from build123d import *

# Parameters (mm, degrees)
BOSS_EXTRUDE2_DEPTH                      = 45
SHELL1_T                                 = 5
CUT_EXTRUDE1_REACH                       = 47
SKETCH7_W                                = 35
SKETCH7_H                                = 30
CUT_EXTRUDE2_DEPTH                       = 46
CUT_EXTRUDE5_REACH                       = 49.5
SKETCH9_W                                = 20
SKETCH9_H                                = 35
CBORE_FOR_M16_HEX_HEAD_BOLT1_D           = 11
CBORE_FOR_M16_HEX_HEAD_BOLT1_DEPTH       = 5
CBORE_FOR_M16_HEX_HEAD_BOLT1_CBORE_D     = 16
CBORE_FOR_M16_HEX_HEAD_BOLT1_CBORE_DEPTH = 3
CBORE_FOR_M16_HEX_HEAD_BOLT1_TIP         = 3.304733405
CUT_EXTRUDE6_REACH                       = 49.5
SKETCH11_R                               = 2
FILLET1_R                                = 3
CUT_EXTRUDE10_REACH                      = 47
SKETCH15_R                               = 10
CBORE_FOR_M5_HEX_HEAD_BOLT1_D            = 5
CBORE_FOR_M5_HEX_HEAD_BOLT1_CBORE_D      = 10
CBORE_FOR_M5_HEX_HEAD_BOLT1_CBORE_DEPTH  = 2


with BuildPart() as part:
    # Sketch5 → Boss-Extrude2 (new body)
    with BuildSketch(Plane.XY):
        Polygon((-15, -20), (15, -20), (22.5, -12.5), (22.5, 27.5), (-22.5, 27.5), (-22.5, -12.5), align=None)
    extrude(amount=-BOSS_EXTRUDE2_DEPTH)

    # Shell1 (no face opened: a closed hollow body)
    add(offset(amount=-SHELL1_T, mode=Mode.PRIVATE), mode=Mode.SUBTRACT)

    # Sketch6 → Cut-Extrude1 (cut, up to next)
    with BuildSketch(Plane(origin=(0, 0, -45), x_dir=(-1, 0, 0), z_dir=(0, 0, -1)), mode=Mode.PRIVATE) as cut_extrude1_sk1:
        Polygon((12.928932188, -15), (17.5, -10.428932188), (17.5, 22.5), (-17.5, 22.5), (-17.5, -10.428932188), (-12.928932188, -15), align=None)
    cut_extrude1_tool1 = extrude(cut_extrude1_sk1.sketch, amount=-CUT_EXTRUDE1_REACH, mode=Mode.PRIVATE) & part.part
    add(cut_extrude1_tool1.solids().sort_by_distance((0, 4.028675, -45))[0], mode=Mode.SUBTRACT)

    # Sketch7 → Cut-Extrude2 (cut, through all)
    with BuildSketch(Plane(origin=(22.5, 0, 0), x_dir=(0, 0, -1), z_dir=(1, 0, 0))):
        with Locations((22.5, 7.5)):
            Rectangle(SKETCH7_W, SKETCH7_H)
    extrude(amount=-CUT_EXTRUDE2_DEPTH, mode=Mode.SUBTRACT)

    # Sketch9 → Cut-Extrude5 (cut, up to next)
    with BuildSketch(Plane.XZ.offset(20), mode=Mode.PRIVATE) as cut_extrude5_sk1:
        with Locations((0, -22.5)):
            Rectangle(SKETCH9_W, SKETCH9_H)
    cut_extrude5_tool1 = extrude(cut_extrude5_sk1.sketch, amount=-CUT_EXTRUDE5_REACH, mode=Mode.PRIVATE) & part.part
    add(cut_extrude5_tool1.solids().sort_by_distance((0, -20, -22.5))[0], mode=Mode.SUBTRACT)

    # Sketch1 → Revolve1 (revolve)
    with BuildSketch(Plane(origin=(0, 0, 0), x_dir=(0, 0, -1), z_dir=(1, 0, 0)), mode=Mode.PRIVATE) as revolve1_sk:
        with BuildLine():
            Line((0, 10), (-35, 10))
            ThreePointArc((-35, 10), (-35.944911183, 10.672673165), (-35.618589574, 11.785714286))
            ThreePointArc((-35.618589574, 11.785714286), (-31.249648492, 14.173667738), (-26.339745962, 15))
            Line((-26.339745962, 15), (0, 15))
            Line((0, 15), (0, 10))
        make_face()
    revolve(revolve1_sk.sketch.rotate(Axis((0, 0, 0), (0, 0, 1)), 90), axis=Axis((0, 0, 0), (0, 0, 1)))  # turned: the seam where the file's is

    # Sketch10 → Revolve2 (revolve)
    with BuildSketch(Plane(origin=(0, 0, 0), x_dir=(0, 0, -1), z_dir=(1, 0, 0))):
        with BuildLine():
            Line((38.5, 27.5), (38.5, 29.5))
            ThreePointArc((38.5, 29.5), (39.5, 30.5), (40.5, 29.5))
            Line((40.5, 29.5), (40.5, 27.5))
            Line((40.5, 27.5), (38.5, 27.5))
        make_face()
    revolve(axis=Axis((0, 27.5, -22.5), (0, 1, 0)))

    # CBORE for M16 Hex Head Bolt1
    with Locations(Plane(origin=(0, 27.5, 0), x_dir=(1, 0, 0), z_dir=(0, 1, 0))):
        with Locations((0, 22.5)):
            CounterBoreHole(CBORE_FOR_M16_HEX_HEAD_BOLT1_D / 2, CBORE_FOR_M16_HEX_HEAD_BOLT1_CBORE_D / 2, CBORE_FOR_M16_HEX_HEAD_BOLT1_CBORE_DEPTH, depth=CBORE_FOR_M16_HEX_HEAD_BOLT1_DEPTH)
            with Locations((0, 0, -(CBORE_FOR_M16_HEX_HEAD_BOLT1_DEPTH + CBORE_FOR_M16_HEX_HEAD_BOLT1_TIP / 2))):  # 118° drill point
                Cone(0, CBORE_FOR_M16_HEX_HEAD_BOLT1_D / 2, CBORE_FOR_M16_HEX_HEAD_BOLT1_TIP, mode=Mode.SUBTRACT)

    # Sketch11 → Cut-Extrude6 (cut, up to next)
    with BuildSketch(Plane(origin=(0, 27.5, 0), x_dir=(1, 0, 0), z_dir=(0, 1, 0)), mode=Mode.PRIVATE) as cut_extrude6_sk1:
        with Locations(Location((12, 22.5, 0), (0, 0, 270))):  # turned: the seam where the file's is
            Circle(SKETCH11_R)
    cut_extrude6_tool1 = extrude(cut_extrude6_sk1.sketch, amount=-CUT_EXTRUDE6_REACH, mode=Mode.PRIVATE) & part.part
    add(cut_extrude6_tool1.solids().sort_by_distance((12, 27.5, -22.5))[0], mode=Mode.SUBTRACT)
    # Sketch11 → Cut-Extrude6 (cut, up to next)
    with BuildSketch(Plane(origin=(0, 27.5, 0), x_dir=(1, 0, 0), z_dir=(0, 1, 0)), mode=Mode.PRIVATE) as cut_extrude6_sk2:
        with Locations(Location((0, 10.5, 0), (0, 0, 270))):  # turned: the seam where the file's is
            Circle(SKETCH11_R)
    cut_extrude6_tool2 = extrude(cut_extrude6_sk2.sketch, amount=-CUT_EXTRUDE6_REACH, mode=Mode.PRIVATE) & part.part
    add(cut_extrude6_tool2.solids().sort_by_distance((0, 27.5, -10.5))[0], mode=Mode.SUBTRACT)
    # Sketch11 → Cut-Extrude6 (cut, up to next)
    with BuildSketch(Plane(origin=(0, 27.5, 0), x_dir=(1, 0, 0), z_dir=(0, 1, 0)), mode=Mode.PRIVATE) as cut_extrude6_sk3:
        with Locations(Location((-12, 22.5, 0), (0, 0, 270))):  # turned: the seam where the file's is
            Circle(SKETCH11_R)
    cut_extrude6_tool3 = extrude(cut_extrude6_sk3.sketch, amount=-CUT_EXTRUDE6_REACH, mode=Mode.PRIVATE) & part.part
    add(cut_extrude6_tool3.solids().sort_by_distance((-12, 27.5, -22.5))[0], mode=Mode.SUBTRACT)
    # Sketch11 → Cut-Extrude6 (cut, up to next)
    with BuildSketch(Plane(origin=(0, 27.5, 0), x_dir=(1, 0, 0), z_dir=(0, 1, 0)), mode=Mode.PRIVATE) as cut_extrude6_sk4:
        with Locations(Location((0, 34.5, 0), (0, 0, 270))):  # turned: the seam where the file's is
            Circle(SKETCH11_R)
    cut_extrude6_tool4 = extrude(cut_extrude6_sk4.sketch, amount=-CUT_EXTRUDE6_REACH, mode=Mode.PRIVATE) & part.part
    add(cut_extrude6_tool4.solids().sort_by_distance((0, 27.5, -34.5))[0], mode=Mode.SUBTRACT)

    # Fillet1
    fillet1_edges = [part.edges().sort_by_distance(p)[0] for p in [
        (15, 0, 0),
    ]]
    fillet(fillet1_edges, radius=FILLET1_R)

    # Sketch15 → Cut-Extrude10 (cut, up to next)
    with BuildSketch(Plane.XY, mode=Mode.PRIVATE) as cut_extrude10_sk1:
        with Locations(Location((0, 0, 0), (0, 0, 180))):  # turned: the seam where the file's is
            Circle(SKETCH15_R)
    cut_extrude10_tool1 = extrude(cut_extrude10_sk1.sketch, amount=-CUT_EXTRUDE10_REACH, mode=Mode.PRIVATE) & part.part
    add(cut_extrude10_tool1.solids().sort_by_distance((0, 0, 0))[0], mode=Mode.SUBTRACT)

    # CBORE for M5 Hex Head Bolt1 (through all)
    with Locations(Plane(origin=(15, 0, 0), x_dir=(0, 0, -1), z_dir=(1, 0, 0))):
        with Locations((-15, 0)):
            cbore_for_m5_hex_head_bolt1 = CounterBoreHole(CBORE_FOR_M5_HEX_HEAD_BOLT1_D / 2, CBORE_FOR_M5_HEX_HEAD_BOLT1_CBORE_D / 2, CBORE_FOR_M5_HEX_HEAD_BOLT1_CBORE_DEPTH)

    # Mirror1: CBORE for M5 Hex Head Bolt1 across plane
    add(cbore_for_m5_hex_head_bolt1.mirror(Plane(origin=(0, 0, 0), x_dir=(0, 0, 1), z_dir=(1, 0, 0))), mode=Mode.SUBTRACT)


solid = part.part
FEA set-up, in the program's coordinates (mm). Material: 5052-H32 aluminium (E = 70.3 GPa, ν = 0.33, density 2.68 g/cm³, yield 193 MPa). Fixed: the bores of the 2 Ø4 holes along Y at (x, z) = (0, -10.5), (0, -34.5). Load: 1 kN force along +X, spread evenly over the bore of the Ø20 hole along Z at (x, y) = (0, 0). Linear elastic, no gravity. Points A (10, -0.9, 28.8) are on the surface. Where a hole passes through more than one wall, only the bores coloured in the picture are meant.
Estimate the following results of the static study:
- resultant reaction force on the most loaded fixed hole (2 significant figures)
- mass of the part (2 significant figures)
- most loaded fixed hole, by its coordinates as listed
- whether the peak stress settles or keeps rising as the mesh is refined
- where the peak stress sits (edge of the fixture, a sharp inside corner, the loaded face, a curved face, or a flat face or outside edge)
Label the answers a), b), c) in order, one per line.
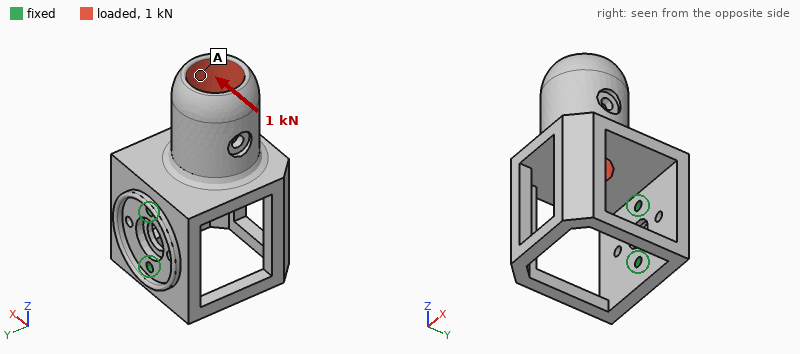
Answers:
a) 1.8 kN
b) 100 g
c) (0, -10.5)
d) keeps rising
e) edge of the fixture
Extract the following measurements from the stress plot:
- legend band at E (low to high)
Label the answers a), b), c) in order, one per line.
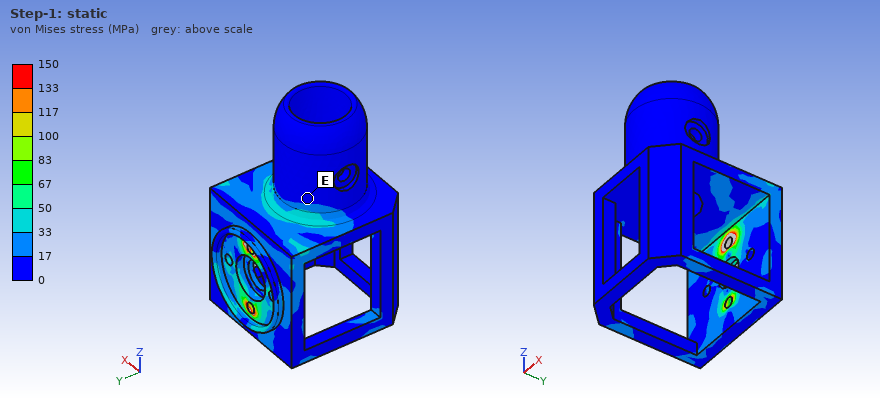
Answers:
a) 0 to 17 MPa
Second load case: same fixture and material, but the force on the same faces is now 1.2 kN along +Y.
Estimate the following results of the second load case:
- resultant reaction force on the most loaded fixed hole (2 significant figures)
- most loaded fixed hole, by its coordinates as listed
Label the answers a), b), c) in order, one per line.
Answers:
a) 1.9 kN
b) (0, -10.5)
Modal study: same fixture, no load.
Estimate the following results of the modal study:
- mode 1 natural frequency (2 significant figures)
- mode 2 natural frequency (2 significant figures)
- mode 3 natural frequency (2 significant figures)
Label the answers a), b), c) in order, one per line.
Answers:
a) 1300 Hz
b) 1300 Hz
c) 2300 Hz
